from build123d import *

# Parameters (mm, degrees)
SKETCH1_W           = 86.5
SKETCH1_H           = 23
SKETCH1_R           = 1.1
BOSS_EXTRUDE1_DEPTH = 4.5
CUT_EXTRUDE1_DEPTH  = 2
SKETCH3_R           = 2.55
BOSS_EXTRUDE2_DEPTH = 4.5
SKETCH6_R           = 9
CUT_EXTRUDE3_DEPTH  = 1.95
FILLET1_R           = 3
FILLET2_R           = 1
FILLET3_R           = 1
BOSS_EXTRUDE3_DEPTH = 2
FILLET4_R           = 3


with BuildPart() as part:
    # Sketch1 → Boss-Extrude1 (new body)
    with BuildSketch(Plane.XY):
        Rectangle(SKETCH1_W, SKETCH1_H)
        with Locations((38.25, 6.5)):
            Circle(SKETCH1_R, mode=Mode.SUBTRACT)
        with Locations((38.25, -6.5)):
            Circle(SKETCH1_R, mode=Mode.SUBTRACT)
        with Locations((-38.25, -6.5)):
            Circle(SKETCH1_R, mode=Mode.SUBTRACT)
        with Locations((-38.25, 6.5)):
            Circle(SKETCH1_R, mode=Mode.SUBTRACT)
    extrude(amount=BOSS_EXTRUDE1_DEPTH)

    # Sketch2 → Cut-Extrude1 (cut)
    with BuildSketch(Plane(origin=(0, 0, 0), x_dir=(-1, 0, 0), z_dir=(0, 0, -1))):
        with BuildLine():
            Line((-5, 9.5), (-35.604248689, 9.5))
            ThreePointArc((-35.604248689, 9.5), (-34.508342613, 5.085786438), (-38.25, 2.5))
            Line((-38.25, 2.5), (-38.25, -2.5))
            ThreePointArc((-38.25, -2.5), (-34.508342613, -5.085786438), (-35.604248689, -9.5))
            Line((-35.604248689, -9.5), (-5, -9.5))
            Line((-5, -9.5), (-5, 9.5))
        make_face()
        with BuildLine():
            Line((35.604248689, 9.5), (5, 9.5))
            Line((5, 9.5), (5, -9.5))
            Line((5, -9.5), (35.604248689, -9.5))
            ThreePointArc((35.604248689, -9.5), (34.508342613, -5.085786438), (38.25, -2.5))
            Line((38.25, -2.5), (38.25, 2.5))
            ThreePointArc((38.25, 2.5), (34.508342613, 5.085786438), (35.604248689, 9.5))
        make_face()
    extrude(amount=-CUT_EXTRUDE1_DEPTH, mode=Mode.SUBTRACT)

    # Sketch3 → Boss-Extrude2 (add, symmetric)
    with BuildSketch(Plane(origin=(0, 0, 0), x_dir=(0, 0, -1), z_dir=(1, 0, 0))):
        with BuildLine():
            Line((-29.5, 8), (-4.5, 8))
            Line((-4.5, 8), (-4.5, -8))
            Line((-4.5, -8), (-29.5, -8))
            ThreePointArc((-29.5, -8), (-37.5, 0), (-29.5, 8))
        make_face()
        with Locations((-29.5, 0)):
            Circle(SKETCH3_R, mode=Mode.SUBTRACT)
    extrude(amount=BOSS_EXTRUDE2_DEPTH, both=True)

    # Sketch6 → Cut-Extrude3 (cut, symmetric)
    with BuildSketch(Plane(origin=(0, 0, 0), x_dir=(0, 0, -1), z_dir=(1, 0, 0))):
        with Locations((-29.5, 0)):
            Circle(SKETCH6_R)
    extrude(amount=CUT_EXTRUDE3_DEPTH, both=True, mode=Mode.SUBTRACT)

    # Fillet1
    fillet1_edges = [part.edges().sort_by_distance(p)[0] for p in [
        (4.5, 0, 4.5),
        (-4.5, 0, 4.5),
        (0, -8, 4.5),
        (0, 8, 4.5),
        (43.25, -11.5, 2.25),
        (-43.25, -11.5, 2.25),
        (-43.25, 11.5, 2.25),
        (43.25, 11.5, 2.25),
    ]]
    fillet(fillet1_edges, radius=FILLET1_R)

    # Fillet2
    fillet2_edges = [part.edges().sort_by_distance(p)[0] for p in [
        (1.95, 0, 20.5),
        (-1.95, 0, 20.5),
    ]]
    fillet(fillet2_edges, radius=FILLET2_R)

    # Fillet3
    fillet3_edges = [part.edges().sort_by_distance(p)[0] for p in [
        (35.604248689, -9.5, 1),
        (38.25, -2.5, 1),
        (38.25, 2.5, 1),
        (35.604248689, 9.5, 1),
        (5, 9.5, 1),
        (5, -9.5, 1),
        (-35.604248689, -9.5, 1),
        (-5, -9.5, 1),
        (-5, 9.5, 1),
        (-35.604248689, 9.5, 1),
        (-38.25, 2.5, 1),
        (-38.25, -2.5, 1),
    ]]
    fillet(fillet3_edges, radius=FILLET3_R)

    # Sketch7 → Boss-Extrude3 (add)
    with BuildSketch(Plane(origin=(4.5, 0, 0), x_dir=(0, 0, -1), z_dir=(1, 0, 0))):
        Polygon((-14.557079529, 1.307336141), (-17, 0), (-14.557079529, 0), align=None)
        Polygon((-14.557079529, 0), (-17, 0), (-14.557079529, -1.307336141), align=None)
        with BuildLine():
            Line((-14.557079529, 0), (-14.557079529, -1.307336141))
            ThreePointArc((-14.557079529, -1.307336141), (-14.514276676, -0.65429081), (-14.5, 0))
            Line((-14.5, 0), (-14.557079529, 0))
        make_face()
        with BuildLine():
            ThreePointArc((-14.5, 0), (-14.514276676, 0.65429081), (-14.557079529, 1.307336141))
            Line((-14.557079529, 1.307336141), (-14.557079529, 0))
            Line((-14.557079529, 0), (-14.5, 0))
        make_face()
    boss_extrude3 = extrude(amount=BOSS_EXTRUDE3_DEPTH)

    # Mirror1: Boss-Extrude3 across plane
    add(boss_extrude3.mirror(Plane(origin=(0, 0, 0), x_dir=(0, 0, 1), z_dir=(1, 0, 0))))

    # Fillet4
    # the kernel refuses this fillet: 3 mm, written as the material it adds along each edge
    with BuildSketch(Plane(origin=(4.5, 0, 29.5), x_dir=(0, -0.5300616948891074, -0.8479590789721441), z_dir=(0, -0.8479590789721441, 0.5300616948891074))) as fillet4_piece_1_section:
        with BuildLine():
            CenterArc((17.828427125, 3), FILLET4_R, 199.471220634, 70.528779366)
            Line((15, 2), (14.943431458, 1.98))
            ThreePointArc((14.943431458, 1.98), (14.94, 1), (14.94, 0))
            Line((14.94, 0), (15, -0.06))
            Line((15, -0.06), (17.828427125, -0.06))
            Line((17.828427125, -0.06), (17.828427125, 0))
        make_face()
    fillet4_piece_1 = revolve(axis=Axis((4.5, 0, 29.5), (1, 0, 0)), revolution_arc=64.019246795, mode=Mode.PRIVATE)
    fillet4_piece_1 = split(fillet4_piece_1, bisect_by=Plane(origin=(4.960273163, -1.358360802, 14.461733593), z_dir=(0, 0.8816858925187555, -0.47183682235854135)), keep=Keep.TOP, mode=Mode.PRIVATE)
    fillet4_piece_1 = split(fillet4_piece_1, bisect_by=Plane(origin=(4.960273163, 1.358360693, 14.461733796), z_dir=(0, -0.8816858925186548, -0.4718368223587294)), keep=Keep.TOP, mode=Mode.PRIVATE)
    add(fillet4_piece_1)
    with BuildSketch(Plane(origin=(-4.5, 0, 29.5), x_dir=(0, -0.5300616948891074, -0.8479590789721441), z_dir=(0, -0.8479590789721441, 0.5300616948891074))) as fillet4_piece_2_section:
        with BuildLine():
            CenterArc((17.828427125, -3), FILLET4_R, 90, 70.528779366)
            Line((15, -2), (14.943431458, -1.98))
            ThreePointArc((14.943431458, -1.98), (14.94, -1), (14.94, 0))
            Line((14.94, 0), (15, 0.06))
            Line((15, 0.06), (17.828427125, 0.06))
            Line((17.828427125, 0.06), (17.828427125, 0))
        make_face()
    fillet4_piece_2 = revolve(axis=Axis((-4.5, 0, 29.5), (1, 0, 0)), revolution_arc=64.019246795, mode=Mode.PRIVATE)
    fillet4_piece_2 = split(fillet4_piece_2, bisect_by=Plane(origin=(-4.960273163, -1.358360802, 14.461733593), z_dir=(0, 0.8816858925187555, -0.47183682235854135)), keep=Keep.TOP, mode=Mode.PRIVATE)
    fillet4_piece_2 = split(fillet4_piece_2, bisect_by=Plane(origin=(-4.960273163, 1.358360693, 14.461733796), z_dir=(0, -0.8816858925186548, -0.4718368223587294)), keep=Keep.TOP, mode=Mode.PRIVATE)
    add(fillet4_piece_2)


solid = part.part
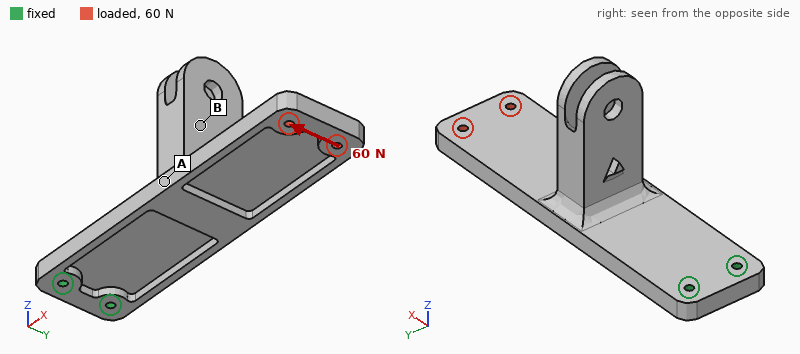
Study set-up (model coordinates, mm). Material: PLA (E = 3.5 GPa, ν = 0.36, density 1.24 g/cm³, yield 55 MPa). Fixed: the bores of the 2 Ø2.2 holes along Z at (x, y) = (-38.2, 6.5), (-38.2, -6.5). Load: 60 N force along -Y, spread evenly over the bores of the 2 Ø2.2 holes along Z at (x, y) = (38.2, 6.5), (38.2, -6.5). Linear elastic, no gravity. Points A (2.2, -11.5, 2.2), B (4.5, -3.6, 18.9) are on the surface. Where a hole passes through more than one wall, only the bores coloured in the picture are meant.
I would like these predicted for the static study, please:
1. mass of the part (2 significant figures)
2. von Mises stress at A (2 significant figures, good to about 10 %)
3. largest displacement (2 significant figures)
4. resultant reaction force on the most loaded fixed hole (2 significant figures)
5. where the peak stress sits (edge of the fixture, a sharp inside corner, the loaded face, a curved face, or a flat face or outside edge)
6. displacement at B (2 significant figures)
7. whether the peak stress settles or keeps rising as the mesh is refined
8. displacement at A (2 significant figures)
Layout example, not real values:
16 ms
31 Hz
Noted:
13 g
6.1 MPa
1.1 mm
320 N
edge of the fixture
0.20 mm
keeps rising
0.40 mm
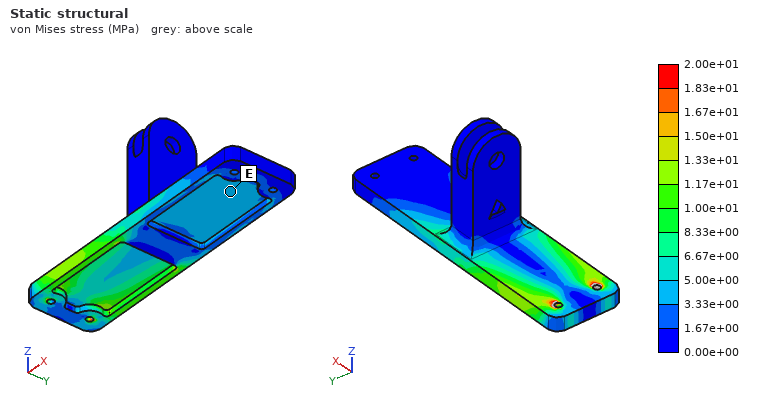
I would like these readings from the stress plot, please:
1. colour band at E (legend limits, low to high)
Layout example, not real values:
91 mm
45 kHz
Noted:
3.33e+00 to 5.00e+00 MPa
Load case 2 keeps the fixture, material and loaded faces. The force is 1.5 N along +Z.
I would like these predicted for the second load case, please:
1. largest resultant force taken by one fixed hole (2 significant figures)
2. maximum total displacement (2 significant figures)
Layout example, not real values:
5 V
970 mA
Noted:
2.1 N
0.90 mm
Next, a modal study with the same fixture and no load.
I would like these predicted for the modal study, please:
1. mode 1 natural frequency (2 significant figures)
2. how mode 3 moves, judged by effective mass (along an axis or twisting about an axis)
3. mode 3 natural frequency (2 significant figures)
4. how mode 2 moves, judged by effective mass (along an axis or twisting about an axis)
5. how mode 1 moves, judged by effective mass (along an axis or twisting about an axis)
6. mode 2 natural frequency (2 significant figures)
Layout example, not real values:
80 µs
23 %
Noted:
120 Hz
along Z
680 Hz
along Y
along Z
400 Hz
